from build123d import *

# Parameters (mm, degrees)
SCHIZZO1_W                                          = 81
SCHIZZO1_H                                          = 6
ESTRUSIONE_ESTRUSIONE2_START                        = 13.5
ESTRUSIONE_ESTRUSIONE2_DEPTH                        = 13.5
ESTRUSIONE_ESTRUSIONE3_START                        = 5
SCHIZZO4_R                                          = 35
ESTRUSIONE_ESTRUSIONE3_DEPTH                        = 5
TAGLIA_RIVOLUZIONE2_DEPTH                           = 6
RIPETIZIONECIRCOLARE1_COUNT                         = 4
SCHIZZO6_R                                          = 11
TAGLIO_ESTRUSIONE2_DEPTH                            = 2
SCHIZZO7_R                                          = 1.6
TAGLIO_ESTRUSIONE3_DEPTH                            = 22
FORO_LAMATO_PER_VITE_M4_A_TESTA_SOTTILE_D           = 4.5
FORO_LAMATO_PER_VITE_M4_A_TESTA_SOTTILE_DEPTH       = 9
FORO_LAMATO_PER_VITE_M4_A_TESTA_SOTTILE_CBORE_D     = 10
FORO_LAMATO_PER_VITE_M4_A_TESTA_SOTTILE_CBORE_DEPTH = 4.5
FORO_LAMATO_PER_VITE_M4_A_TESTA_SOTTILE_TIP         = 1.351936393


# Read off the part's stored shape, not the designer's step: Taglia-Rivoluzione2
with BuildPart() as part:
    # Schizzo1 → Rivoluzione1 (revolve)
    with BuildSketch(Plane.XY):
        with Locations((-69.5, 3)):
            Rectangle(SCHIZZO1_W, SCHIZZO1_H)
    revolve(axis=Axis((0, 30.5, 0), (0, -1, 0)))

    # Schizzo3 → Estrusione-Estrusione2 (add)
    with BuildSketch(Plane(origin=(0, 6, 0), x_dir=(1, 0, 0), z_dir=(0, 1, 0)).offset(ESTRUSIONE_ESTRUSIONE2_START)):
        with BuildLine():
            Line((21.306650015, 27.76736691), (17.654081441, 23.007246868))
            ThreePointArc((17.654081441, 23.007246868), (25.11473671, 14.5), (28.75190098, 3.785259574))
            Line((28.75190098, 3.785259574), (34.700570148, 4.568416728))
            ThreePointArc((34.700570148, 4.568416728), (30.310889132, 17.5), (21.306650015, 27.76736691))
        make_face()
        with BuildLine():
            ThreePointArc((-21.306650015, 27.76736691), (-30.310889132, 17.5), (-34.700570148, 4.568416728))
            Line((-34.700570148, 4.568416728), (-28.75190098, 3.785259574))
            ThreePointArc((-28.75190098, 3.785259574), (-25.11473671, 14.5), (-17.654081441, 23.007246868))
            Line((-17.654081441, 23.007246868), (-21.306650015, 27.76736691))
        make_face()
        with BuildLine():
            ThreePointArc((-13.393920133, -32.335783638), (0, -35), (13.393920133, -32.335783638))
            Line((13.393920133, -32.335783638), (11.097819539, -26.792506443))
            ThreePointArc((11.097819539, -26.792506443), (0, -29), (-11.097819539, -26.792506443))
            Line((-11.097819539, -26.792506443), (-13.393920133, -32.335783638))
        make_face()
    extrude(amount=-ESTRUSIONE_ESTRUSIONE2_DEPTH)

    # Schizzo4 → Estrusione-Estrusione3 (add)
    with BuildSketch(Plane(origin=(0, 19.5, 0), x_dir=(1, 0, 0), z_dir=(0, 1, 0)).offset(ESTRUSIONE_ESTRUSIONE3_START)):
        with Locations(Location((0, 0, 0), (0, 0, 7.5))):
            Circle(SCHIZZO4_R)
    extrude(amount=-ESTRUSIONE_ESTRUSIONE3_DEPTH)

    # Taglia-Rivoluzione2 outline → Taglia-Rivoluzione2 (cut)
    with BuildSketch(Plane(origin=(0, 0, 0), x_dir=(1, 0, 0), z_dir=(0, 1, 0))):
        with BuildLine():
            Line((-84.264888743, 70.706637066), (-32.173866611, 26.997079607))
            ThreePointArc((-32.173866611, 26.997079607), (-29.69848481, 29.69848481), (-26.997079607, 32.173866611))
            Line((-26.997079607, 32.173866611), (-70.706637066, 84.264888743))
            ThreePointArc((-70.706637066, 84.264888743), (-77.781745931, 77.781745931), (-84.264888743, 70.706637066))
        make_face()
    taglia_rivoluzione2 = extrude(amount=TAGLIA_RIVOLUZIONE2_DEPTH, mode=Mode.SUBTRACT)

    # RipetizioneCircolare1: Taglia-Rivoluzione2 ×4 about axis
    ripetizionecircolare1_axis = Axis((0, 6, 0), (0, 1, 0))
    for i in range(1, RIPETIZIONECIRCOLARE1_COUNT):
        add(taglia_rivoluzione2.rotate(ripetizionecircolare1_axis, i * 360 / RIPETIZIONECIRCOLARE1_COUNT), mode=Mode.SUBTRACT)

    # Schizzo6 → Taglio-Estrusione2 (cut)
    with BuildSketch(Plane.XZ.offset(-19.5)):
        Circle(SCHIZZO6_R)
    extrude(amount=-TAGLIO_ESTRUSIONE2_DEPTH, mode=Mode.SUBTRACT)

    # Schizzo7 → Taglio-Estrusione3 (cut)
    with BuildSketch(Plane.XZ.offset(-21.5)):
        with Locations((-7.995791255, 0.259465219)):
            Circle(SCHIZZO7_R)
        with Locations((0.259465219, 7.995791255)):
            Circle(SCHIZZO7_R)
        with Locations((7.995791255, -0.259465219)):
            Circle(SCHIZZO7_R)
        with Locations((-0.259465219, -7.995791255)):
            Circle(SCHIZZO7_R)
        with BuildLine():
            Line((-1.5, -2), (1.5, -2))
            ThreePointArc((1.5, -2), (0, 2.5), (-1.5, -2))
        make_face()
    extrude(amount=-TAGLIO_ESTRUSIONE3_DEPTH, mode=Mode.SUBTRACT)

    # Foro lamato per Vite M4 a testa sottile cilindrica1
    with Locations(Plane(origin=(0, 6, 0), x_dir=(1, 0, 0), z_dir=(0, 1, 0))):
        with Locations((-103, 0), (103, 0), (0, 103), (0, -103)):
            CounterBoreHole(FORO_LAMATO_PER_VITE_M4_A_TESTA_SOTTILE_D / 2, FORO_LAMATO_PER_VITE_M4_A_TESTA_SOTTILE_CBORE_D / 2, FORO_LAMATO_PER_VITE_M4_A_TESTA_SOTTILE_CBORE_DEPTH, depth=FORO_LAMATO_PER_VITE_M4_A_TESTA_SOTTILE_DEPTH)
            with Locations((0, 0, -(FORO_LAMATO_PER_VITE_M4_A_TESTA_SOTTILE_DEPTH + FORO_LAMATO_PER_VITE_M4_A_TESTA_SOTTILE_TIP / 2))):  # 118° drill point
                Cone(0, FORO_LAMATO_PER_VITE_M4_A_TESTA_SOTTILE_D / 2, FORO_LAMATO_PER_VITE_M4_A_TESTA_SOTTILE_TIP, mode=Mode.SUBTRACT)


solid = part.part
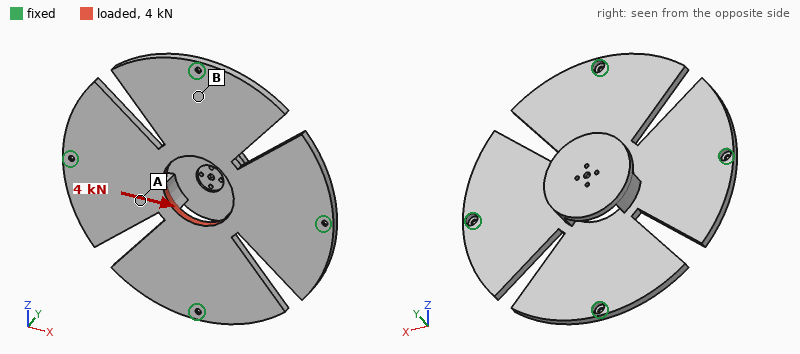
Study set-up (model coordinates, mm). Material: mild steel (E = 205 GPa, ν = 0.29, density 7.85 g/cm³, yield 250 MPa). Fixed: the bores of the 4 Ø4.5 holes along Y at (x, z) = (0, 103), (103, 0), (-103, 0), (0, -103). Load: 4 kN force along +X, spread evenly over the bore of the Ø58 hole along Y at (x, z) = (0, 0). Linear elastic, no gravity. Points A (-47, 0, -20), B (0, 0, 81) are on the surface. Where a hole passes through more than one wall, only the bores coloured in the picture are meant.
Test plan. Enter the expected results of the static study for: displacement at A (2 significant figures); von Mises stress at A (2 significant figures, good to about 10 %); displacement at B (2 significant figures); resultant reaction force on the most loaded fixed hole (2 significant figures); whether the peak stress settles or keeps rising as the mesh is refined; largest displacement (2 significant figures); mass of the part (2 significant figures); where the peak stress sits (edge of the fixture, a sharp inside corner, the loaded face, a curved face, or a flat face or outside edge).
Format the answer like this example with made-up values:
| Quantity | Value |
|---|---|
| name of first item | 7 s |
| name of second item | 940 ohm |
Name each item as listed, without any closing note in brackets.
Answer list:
| Quantity | Value |
|---|---|
| displacement at A | 8.3 µm |
| von Mises stress at A | 8.3 MPa |
| displacement at B | 2.2 µm |
| resultant reaction force on the most loaded fixed hole | 1.7 kN |
| whether the peak stress settles or keeps rising as the mesh is refined | keeps rising |
| largest displacement | 10 µm |
| mass of the part | 1.7 kg |
| where the peak stress sits | edge of the fixture |
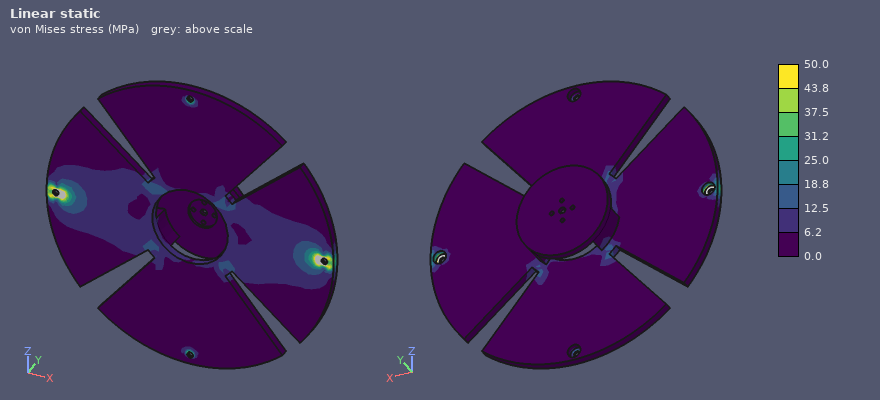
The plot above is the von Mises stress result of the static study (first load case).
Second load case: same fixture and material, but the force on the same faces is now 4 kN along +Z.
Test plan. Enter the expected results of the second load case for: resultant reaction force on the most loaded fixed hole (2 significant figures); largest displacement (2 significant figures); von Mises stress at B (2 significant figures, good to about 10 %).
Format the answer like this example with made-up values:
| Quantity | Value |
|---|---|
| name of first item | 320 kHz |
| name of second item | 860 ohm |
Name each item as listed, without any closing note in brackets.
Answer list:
| Quantity | Value |
|---|---|
| resultant reaction force on the most loaded fixed hole | 1.8 kN |
| largest displacement | 9.9 µm |
| von Mises stress at B | 13 MPa |
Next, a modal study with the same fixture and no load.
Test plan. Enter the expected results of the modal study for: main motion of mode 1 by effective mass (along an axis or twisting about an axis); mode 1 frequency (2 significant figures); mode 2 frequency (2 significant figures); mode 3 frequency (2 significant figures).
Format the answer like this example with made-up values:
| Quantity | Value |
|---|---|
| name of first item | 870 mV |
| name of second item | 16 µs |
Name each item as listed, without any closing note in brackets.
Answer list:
| Quantity | Value |
|---|---|
| main motion of mode 1 by effective mass | along Y |
| mode 1 frequency | 560 Hz |
| mode 2 frequency | 720 Hz |
| mode 3 frequency | 720 Hz |
